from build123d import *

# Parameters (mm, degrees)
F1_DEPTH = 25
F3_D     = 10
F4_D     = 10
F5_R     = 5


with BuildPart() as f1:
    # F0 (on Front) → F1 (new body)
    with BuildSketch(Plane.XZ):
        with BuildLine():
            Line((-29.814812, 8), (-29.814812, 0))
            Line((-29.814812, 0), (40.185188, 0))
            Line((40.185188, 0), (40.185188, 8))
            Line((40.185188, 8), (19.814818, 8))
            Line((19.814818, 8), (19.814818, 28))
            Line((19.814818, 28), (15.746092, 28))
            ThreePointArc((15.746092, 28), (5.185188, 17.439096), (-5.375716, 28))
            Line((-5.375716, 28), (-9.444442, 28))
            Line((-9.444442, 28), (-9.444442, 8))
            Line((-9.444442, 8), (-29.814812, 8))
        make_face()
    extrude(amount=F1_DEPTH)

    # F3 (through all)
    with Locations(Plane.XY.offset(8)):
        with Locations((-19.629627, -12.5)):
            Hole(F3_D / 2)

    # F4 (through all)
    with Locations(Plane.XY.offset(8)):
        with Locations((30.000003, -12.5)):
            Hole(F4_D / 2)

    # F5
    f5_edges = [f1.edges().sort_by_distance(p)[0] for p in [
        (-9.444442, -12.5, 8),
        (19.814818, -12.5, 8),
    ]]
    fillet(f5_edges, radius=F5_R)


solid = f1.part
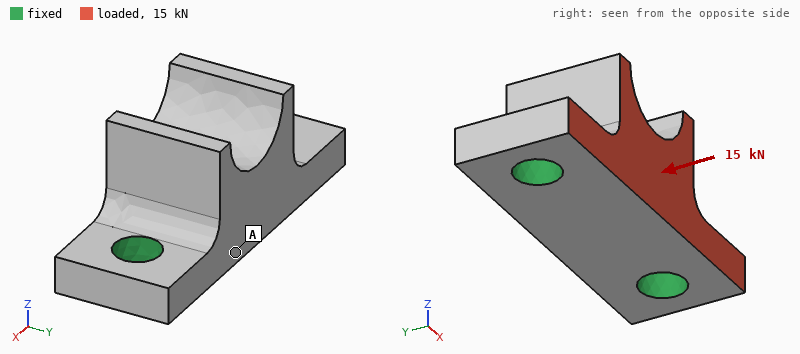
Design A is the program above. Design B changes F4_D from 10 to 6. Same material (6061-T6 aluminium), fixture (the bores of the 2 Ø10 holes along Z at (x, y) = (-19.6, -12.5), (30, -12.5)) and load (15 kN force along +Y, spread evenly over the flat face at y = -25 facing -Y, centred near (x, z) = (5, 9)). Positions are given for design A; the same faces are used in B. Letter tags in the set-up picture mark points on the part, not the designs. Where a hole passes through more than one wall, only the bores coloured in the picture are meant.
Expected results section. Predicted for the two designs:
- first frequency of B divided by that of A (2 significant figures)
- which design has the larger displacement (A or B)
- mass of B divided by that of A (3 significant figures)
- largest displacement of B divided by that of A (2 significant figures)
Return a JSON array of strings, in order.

["0.91", "B", "1.02", "1.2"]
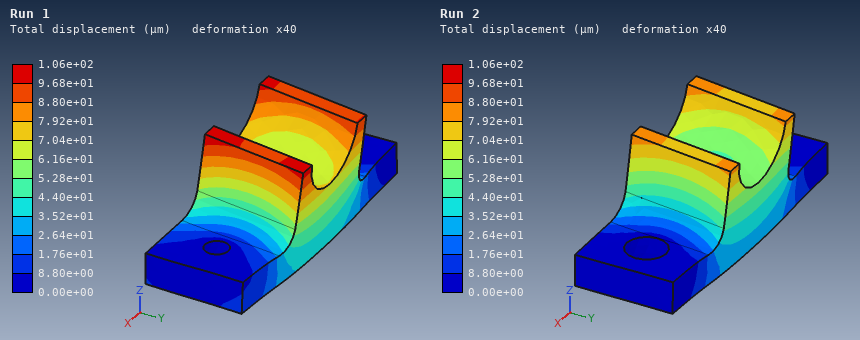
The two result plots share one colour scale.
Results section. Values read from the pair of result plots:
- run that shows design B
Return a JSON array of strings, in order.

["Run 1"]
